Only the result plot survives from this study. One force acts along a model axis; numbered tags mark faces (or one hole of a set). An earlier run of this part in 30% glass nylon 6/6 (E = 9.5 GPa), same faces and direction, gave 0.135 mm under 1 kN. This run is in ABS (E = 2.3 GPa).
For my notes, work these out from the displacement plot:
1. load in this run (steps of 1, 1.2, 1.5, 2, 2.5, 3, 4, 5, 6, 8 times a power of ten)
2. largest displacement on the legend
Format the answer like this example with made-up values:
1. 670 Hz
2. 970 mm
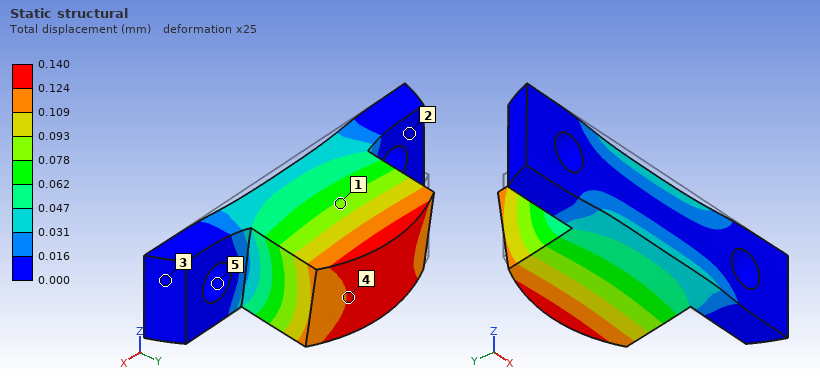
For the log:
1. 250 N
2. 0.140 mm
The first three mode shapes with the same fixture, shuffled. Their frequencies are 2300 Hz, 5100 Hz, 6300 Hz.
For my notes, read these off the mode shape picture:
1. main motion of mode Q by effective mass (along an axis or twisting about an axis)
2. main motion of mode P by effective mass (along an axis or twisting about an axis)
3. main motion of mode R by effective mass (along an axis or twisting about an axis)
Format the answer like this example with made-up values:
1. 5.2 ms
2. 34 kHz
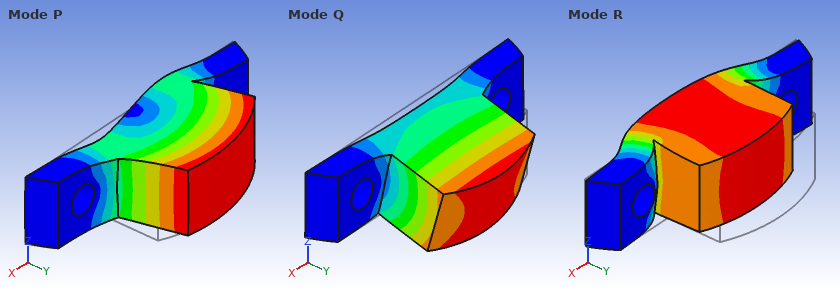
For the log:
1. along Z
2. along X
3. along Y
